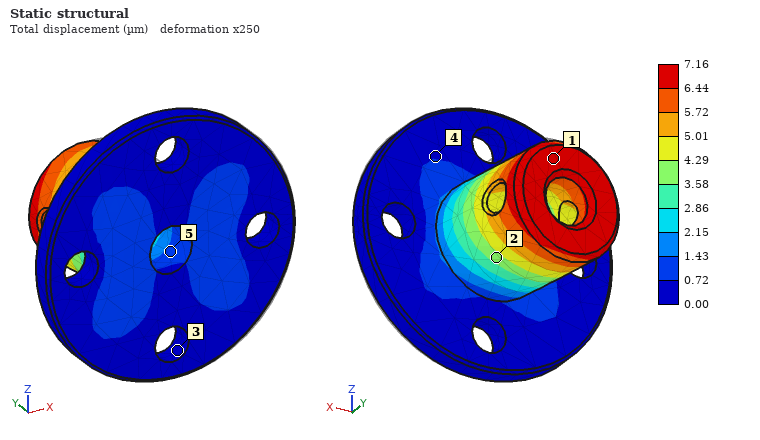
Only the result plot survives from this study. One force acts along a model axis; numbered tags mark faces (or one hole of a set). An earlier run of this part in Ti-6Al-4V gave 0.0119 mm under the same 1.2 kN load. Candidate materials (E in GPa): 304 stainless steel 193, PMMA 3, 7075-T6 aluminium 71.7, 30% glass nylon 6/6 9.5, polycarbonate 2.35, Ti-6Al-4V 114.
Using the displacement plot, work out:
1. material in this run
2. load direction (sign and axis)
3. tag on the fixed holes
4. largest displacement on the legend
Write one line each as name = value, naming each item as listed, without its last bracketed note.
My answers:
material in this run = 304 stainless steel
load direction = -X
tag on the fixed holes = 3
largest displacement on the legend = 7.16 µm
